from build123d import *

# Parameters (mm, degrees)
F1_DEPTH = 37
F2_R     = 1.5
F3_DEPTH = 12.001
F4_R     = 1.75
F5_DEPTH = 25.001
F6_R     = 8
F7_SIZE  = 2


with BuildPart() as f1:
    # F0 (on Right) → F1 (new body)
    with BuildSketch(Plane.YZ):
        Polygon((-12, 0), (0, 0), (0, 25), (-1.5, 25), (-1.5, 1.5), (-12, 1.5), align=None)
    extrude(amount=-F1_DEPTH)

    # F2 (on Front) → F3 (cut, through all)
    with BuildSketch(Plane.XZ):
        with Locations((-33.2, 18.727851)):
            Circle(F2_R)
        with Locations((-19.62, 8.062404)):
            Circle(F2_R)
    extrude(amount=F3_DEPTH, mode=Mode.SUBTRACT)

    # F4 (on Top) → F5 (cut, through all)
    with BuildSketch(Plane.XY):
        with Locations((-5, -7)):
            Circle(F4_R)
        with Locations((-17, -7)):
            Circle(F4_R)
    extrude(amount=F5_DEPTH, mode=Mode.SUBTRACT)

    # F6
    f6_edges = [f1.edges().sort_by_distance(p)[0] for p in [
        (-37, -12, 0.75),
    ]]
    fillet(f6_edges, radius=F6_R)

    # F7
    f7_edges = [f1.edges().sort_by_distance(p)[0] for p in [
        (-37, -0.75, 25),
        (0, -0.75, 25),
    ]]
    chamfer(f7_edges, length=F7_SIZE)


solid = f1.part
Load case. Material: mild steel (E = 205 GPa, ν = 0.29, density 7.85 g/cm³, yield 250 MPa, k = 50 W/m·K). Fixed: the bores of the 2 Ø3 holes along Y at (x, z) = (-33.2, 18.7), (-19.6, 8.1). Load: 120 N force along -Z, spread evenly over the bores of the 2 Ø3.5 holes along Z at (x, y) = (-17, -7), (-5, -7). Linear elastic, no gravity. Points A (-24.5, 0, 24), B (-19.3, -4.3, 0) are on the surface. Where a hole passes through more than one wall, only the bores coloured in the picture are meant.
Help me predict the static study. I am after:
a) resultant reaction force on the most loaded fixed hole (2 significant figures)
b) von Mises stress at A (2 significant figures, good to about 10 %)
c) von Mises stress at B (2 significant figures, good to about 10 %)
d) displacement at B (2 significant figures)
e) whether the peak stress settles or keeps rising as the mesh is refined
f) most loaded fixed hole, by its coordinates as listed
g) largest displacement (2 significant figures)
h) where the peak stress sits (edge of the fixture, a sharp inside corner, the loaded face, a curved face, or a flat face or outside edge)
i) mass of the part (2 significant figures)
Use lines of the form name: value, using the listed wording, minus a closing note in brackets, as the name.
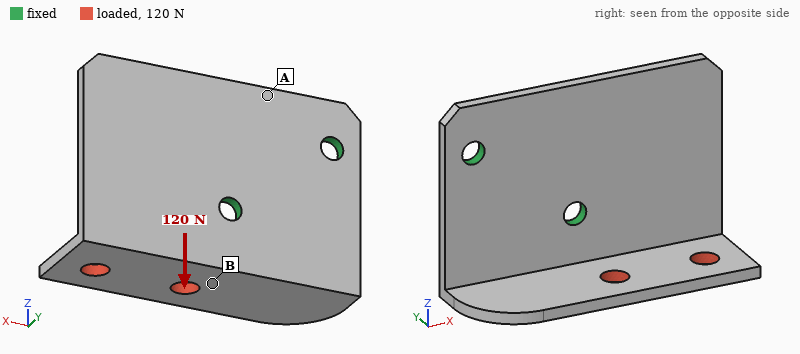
resultant reaction force on the most loaded fixed hole: 150 N
von Mises stress at A: 17 MPa
von Mises stress at B: 39 MPa
displacement at B: 20 µm
whether the peak stress settles or keeps rising as the mesh is refined: keeps rising
most loaded fixed hole, by its coordinates as listed: (-19.6, 8.1)
largest displacement: 69 µm
where the peak stress sits: edge of the fixture
mass of the part: 15 g
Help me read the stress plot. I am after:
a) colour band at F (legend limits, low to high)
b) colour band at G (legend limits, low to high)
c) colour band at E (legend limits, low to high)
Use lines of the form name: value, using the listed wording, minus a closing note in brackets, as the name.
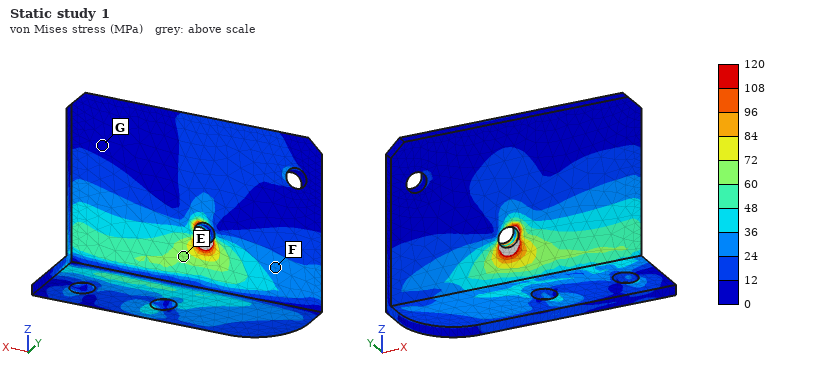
colour band at F: 24 to 36 MPa
colour band at G: 0 to 12 MPa
colour band at E: 60 to 72 MPa
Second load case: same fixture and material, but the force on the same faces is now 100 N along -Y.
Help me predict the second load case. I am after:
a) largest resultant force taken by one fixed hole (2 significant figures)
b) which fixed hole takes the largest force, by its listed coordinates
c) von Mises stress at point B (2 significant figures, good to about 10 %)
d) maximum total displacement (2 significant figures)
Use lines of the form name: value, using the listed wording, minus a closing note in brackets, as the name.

largest resultant force taken by one fixed hole: 130 N
which fixed hole takes the largest force, by its listed coordinates: (-19.6, 8.1)
von Mises stress at point B: 23 MPa
maximum total displacement: 58 µm
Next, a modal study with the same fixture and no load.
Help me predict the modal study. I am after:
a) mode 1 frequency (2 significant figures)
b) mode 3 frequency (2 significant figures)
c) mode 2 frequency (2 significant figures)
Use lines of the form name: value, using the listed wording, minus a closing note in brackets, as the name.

mode 1 frequency: 2900 Hz
mode 3 frequency: 4800 Hz
mode 2 frequency: 3700 Hz
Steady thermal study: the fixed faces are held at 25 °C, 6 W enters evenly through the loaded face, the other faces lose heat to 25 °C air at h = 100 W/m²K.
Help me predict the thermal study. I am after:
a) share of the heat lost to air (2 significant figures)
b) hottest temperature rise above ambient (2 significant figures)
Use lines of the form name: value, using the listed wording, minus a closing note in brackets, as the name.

share of the heat lost to air: 53 %
hottest temperature rise above ambient: 44 K
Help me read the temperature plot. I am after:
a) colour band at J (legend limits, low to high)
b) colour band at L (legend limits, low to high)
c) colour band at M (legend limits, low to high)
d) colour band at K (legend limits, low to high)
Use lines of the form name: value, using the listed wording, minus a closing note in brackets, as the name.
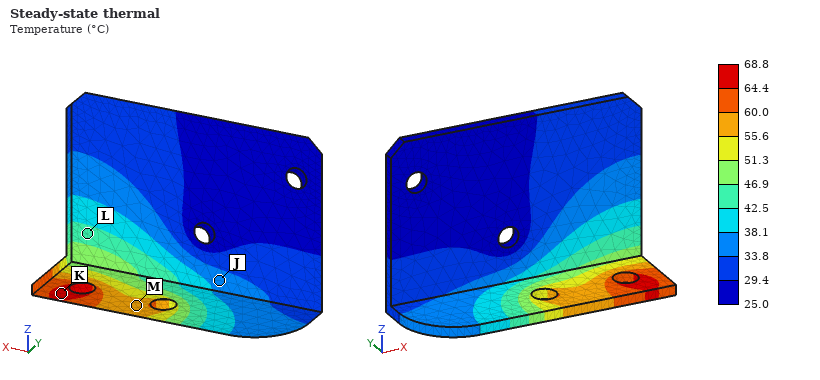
colour band at J: 33.8 to 38.1 °C
colour band at L: 42.5 to 46.9 °C
colour band at M: 55.6 to 60.0 °C
colour band at K: 64.4 to 68.8 °C
